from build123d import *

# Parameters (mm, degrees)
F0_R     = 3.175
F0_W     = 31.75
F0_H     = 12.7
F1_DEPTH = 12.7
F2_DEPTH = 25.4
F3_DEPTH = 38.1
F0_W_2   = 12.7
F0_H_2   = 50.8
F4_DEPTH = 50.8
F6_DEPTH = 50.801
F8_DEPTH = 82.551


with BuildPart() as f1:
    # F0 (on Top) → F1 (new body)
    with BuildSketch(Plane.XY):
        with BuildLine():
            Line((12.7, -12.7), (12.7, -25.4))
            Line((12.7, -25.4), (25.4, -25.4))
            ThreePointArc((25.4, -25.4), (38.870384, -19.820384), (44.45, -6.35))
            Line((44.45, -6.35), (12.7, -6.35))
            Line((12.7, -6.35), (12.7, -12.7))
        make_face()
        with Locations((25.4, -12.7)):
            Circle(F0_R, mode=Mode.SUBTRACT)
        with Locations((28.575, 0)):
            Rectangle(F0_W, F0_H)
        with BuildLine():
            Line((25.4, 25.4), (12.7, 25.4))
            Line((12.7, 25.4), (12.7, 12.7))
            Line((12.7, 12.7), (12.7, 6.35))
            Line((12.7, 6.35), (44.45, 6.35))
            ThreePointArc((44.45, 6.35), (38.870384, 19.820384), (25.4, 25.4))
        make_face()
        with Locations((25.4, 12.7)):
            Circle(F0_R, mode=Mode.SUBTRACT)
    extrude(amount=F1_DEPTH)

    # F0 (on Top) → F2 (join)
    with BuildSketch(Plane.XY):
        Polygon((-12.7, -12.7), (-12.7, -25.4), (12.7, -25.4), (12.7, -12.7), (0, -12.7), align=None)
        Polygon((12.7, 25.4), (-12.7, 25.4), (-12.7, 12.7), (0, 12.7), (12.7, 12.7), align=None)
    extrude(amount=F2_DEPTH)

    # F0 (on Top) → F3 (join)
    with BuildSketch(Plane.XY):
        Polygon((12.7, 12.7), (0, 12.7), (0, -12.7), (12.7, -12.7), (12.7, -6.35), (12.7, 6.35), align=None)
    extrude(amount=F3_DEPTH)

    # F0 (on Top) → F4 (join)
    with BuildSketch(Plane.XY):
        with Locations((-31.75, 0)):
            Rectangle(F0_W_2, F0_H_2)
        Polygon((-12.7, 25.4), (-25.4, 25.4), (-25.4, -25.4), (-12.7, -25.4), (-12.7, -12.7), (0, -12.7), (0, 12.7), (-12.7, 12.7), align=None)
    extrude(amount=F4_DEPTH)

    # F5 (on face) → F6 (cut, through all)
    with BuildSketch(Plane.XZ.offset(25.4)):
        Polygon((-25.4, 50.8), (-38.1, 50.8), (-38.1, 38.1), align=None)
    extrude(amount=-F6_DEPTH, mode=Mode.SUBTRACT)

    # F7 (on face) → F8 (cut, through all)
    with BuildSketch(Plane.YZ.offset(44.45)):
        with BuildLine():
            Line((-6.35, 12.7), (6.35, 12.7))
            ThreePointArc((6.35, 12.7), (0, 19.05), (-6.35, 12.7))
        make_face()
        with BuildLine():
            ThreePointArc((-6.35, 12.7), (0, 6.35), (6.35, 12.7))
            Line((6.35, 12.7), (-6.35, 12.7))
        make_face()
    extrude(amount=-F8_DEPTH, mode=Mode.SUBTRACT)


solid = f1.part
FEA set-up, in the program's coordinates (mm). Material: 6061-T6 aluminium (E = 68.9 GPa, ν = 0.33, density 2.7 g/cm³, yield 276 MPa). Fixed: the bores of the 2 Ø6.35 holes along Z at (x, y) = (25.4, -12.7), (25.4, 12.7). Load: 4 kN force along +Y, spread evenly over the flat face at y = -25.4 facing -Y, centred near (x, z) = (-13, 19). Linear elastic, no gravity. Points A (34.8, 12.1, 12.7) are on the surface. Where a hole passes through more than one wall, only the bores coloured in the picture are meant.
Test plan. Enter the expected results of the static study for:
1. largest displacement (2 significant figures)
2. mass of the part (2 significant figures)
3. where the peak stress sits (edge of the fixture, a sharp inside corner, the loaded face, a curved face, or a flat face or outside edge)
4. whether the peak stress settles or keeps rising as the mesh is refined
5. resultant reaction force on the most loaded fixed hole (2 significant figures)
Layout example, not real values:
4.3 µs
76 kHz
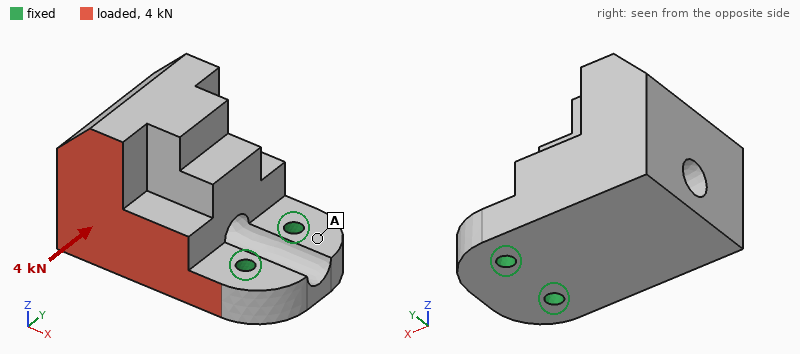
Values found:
53 µm
310 g
edge of the fixture
keeps rising
5.5 kN
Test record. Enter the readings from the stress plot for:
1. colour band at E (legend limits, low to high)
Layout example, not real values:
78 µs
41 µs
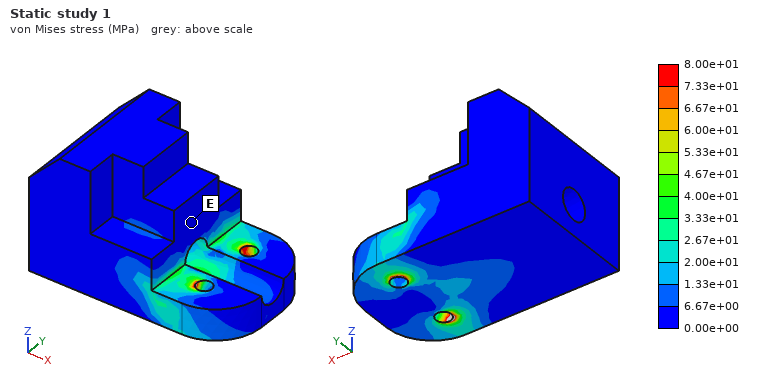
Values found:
0.00e+00 to 6.67e+00 MPa
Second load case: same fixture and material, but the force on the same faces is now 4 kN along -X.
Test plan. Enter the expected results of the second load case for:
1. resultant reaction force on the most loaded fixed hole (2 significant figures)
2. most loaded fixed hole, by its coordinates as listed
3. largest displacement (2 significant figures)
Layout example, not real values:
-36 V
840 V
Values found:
5.5 kN
(25.4, -12.7)
0.13 mm
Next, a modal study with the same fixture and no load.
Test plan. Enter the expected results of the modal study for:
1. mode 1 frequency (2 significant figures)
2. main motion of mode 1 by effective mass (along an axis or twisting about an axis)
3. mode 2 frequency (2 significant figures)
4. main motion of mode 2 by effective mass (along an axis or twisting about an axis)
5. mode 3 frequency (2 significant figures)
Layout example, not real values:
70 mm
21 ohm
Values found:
1200 Hz
along Z
2900 Hz
along Y
5100 Hz
